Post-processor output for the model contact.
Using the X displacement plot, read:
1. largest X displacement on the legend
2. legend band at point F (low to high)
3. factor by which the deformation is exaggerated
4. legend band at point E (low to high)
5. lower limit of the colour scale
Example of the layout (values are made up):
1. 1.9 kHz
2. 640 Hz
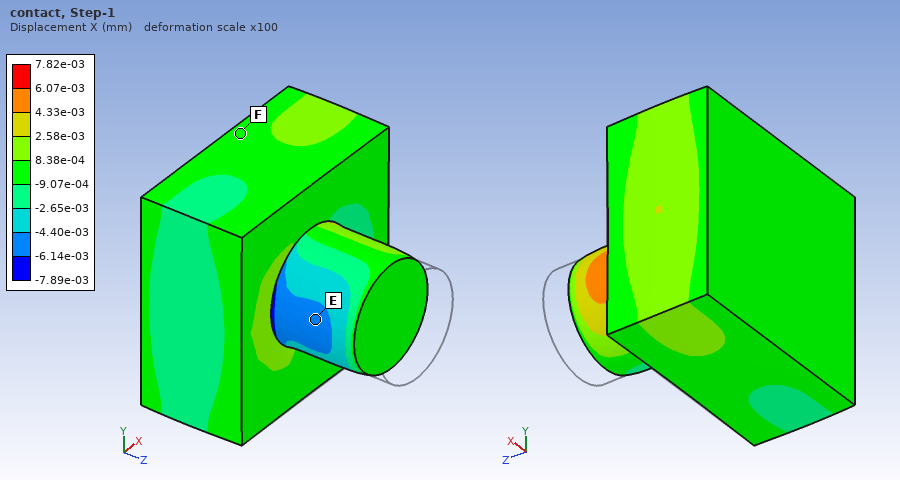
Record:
1. 7.82e-03 mm
2. -9.07e-04 to 8.38e-04 mm
3. 100
4. -6.14e-03 to -4.40e-03 mm
5. -7.89e-03 mm
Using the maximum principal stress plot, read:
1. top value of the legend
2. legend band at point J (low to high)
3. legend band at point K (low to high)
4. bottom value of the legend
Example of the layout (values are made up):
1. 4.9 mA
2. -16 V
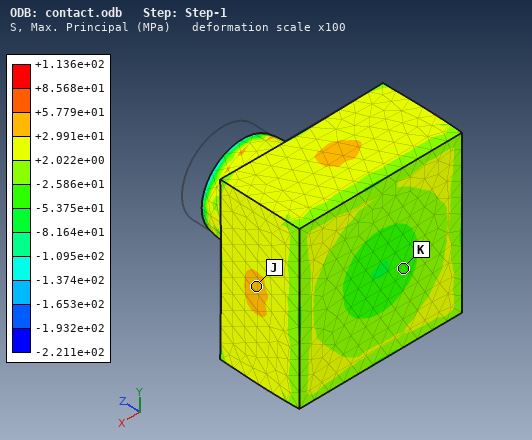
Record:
1. +1.136e+02 MPa
2. +2.991e+01 to +5.779e+01 MPa
3. -5.375e+01 to -2.586e+01 MPa
4. -2.211e+02 MPa
